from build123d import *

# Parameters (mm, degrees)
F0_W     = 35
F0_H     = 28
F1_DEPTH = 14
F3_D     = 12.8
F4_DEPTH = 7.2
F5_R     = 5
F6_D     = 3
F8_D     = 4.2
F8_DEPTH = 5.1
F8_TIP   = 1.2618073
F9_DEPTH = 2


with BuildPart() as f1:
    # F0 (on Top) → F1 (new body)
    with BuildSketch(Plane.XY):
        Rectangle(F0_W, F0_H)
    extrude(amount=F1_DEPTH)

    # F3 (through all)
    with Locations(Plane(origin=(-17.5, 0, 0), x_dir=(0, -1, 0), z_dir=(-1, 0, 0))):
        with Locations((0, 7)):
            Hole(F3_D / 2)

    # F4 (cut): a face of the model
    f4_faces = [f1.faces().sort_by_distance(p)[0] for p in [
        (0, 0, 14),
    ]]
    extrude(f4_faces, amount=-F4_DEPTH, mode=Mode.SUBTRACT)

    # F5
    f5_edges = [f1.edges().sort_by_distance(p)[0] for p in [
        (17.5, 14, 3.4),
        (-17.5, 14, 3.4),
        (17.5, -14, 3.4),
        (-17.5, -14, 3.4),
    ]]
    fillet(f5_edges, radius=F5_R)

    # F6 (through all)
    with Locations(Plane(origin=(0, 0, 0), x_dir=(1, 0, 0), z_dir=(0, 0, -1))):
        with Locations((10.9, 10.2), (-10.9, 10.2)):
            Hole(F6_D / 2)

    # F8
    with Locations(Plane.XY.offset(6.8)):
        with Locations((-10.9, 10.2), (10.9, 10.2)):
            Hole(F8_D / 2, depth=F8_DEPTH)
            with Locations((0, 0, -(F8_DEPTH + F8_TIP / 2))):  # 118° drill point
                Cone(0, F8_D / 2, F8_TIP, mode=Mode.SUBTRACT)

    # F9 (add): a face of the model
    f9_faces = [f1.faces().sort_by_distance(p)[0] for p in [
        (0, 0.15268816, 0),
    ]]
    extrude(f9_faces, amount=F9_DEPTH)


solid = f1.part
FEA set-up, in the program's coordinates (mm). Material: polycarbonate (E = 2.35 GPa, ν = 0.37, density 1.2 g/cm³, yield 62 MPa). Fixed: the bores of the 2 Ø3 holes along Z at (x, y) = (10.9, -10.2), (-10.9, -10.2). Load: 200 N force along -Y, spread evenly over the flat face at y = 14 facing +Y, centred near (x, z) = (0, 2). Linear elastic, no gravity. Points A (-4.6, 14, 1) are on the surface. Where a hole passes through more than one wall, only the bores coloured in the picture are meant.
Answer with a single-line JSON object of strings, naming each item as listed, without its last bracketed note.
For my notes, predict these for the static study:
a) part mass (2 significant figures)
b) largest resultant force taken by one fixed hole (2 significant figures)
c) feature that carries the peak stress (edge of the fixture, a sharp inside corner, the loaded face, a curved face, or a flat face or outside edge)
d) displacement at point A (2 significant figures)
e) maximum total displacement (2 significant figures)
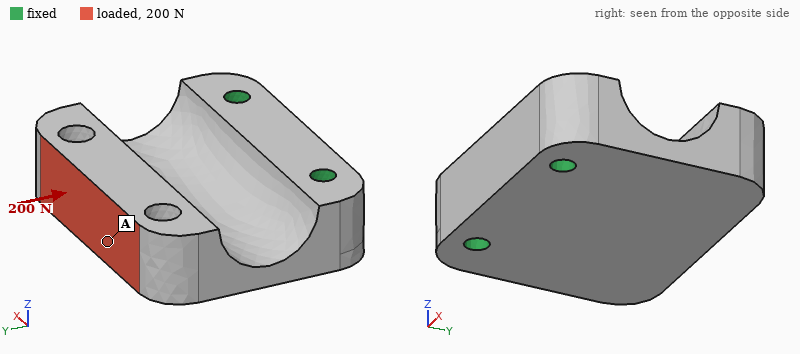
{"part mass": "7.2 g", "largest resultant force taken by one fixed hole": "100 N", "feature that carries the peak stress": "a curved face", "displacement at point A": "0.43 mm", "maximum total displacement": "0.49 mm"}
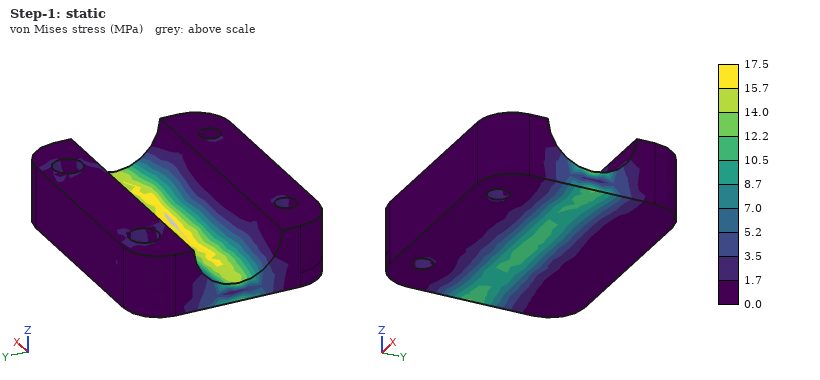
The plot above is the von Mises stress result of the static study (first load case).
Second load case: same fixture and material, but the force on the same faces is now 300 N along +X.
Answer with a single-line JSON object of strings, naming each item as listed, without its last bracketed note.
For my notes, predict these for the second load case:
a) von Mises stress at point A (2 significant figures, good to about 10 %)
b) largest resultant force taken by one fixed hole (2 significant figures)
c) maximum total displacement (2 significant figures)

{"von Mises stress at point A": "2.6 MPa", "largest resultant force taken by one fixed hole": "330 N", "maximum total displacement": "0.21 mm"}
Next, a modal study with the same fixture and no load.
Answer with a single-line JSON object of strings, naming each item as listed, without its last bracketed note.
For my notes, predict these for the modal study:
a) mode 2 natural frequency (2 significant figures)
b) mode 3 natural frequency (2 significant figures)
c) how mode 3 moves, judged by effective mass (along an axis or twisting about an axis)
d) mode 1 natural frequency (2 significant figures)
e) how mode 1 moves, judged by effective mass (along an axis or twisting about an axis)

{"mode 2 natural frequency": "2800 Hz", "mode 3 natural frequency": "4800 Hz", "how mode 3 moves, judged by effective mass": "along X", "mode 1 natural frequency": "1100 Hz", "how mode 1 moves, judged by effective mass": "along Z"}
